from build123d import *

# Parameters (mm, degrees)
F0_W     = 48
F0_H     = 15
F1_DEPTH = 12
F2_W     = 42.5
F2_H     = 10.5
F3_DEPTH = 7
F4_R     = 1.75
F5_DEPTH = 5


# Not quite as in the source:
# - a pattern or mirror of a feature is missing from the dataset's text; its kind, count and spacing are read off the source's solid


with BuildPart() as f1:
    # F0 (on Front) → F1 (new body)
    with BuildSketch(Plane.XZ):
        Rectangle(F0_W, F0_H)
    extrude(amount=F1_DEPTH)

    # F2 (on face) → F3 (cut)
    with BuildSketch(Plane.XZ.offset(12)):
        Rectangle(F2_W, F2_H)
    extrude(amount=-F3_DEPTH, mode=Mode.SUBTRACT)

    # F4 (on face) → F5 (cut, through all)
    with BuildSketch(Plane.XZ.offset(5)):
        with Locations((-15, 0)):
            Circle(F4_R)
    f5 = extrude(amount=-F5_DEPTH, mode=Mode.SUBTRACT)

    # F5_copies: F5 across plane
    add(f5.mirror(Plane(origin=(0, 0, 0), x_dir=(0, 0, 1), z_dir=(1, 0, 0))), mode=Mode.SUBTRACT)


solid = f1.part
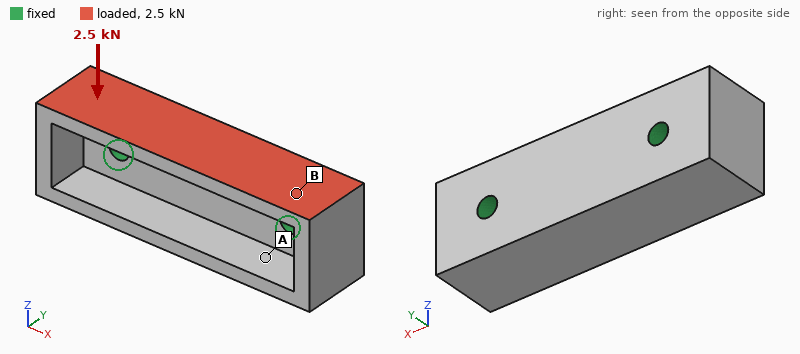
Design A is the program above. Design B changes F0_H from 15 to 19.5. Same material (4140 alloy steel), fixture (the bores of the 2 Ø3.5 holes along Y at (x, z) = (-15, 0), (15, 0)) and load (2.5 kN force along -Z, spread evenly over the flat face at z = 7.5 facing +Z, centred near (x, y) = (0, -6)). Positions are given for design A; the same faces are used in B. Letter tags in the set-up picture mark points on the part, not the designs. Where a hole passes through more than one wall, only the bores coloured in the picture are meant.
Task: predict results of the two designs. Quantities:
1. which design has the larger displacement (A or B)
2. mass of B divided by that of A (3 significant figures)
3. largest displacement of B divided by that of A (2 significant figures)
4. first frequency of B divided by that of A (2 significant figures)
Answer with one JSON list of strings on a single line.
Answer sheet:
["A", "1.48", "0.52", "0.74"]
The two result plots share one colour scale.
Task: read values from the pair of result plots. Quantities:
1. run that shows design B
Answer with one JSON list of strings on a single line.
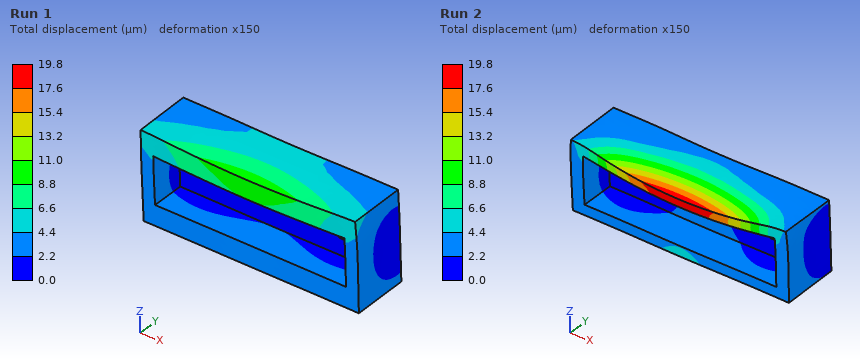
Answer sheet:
["Run 1"]
